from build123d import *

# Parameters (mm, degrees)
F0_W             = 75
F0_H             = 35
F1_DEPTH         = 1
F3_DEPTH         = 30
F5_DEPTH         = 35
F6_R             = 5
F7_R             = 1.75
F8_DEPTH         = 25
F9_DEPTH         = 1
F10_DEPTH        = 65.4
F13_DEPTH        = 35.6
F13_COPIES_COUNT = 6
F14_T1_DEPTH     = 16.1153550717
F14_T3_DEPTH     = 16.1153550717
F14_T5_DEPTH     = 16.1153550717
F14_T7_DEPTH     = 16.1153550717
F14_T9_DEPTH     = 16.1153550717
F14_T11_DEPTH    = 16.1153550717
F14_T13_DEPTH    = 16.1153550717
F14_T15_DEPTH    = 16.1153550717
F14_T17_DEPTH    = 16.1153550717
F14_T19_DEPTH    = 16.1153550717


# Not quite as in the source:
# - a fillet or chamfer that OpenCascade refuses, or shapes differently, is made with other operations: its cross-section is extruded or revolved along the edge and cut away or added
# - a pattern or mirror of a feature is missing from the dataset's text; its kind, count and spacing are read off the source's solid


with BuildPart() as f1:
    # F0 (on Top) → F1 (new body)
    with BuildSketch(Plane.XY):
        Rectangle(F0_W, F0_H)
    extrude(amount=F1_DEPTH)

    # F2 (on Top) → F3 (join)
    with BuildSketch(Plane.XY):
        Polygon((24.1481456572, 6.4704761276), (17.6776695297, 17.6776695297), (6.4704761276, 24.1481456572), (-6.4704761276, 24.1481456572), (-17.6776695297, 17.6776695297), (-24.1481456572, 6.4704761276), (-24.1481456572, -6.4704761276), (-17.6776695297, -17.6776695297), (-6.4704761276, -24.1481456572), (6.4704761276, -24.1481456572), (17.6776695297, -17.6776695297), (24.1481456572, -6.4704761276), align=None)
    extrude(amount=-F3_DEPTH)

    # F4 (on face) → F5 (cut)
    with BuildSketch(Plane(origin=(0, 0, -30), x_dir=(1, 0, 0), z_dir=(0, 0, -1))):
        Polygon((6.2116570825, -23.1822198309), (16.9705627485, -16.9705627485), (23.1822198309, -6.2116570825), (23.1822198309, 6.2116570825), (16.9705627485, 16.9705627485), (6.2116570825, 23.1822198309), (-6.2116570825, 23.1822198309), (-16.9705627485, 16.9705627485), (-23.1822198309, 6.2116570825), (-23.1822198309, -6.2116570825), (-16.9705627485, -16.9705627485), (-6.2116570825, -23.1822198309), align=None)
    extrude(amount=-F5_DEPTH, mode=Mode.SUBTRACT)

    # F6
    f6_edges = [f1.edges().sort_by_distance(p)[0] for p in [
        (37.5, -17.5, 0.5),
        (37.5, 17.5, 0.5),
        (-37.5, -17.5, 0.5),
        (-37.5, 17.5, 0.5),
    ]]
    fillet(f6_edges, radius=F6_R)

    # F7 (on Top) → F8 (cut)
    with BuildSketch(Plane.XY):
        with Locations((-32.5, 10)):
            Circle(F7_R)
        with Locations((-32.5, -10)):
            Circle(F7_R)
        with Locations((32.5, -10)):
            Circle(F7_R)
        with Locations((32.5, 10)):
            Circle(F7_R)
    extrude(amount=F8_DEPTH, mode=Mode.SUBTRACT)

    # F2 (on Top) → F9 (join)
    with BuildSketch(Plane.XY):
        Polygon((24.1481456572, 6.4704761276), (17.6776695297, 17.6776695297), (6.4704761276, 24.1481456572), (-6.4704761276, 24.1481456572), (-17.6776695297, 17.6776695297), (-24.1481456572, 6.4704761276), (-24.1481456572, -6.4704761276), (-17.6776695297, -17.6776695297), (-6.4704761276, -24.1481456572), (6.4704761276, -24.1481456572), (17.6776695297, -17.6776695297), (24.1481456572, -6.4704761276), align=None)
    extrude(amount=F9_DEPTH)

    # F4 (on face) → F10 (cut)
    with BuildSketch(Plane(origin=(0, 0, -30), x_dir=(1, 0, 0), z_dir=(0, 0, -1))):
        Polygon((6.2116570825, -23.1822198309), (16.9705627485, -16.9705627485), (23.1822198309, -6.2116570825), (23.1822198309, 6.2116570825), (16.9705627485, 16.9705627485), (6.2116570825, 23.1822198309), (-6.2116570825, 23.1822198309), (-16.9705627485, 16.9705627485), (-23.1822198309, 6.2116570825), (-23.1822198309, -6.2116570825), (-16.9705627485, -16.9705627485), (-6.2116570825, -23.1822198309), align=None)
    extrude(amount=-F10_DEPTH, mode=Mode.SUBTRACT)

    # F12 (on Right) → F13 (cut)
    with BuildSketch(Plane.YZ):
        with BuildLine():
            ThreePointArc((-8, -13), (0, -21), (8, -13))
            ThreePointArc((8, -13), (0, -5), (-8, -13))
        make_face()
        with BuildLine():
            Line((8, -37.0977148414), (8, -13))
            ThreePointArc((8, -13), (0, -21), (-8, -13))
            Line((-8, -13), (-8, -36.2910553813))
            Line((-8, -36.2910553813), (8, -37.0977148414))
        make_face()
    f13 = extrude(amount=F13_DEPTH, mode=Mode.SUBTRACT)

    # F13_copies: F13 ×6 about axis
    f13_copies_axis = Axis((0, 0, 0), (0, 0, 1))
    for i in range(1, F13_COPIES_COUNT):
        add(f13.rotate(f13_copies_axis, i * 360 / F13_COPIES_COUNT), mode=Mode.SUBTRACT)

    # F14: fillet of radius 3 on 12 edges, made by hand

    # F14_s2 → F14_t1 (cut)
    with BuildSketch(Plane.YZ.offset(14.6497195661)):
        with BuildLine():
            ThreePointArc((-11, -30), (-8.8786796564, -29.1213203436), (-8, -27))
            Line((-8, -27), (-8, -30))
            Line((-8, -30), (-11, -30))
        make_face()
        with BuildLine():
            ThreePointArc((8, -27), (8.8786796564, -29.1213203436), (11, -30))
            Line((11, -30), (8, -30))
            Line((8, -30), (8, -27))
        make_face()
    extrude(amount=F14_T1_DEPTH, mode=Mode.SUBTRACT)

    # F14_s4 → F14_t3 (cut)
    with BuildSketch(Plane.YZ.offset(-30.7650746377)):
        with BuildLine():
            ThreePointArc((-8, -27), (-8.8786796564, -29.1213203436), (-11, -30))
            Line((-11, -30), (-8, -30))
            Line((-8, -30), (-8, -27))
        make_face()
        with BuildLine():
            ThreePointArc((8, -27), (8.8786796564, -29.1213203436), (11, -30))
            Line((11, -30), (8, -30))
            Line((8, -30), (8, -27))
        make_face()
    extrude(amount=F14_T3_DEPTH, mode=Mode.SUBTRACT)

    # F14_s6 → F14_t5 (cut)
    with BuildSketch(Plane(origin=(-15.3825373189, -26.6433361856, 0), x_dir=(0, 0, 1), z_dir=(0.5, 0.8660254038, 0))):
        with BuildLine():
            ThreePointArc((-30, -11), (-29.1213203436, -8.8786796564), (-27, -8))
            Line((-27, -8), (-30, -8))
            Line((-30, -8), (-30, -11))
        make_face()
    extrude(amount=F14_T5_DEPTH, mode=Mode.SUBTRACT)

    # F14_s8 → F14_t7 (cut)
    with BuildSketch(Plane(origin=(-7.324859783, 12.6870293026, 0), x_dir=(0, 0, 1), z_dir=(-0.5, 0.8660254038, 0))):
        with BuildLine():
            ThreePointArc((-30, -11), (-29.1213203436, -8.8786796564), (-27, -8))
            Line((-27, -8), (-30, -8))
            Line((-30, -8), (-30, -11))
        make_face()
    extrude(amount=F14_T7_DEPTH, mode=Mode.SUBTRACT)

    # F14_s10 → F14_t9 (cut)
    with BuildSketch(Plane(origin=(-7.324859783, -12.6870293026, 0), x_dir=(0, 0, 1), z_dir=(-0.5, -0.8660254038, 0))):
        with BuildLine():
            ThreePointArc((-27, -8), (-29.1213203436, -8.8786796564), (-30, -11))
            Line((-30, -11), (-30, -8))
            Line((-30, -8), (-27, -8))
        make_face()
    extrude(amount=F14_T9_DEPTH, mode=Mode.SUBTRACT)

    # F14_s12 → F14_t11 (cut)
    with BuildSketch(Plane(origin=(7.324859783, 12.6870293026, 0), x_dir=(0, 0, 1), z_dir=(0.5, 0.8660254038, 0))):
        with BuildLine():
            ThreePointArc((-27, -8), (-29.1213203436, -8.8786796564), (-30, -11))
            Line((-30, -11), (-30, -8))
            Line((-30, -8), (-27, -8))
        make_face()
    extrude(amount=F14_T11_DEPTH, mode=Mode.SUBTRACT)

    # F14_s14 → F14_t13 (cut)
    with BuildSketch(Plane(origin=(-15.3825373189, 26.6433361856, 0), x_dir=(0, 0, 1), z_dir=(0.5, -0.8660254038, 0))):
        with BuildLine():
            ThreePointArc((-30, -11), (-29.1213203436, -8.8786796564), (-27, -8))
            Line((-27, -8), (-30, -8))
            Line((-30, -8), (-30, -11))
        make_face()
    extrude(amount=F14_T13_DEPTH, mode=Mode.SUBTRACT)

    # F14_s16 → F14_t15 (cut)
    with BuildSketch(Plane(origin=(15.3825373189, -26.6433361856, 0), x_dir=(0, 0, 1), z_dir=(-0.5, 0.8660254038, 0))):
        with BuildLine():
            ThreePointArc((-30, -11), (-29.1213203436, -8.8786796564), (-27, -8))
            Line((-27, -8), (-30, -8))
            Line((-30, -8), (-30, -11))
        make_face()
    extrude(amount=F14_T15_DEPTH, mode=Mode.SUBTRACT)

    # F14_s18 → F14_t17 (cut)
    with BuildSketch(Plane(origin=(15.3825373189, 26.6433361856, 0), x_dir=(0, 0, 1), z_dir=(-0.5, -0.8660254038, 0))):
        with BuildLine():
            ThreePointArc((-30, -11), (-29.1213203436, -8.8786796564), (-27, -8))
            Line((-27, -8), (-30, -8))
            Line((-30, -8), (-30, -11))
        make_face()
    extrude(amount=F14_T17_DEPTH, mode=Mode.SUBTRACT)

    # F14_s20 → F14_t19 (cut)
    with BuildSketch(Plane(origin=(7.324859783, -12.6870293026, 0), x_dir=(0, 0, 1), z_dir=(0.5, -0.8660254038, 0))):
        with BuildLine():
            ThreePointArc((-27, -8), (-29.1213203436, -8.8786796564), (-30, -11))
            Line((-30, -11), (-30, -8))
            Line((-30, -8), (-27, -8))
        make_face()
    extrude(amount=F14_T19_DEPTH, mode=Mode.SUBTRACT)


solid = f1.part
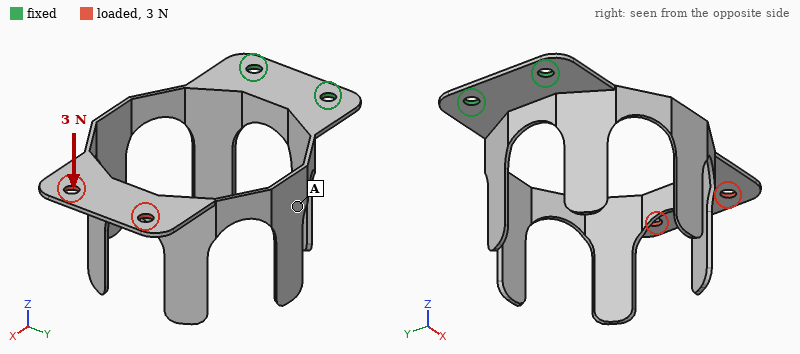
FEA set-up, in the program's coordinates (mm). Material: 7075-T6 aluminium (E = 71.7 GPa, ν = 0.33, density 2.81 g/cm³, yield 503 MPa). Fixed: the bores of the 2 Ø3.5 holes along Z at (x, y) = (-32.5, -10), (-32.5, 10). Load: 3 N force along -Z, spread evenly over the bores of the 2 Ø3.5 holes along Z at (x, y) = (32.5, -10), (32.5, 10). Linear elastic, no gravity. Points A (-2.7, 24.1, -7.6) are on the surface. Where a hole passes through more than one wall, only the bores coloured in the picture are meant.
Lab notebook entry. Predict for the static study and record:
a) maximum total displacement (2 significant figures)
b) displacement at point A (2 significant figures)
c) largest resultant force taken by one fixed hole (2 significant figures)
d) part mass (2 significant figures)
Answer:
1.1 mm
0.29 mm
2.7 N
9.3 g
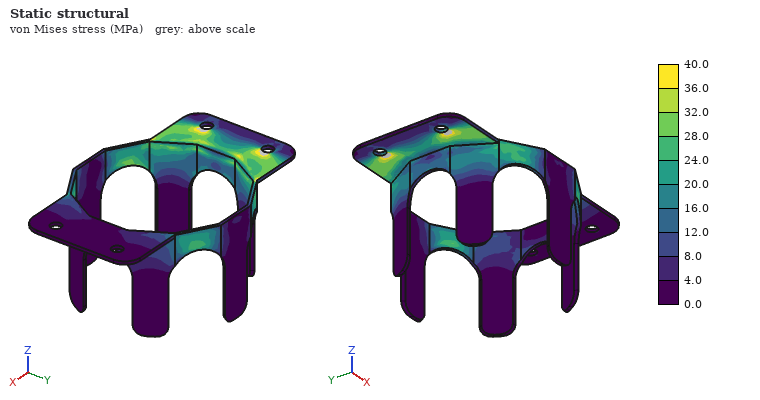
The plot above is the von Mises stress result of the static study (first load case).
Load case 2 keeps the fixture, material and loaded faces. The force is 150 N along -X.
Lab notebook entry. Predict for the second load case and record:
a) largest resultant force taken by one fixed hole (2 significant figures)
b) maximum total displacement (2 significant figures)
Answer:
94 N
0.86 mm
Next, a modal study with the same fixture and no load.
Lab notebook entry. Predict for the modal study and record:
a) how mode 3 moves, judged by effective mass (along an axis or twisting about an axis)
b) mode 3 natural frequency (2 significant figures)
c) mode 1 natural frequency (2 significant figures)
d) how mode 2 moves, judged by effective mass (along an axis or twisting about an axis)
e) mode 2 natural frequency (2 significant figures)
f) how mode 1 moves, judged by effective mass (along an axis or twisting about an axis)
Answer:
twisting about X
480 Hz
160 Hz
along Y
280 Hz
along Z
